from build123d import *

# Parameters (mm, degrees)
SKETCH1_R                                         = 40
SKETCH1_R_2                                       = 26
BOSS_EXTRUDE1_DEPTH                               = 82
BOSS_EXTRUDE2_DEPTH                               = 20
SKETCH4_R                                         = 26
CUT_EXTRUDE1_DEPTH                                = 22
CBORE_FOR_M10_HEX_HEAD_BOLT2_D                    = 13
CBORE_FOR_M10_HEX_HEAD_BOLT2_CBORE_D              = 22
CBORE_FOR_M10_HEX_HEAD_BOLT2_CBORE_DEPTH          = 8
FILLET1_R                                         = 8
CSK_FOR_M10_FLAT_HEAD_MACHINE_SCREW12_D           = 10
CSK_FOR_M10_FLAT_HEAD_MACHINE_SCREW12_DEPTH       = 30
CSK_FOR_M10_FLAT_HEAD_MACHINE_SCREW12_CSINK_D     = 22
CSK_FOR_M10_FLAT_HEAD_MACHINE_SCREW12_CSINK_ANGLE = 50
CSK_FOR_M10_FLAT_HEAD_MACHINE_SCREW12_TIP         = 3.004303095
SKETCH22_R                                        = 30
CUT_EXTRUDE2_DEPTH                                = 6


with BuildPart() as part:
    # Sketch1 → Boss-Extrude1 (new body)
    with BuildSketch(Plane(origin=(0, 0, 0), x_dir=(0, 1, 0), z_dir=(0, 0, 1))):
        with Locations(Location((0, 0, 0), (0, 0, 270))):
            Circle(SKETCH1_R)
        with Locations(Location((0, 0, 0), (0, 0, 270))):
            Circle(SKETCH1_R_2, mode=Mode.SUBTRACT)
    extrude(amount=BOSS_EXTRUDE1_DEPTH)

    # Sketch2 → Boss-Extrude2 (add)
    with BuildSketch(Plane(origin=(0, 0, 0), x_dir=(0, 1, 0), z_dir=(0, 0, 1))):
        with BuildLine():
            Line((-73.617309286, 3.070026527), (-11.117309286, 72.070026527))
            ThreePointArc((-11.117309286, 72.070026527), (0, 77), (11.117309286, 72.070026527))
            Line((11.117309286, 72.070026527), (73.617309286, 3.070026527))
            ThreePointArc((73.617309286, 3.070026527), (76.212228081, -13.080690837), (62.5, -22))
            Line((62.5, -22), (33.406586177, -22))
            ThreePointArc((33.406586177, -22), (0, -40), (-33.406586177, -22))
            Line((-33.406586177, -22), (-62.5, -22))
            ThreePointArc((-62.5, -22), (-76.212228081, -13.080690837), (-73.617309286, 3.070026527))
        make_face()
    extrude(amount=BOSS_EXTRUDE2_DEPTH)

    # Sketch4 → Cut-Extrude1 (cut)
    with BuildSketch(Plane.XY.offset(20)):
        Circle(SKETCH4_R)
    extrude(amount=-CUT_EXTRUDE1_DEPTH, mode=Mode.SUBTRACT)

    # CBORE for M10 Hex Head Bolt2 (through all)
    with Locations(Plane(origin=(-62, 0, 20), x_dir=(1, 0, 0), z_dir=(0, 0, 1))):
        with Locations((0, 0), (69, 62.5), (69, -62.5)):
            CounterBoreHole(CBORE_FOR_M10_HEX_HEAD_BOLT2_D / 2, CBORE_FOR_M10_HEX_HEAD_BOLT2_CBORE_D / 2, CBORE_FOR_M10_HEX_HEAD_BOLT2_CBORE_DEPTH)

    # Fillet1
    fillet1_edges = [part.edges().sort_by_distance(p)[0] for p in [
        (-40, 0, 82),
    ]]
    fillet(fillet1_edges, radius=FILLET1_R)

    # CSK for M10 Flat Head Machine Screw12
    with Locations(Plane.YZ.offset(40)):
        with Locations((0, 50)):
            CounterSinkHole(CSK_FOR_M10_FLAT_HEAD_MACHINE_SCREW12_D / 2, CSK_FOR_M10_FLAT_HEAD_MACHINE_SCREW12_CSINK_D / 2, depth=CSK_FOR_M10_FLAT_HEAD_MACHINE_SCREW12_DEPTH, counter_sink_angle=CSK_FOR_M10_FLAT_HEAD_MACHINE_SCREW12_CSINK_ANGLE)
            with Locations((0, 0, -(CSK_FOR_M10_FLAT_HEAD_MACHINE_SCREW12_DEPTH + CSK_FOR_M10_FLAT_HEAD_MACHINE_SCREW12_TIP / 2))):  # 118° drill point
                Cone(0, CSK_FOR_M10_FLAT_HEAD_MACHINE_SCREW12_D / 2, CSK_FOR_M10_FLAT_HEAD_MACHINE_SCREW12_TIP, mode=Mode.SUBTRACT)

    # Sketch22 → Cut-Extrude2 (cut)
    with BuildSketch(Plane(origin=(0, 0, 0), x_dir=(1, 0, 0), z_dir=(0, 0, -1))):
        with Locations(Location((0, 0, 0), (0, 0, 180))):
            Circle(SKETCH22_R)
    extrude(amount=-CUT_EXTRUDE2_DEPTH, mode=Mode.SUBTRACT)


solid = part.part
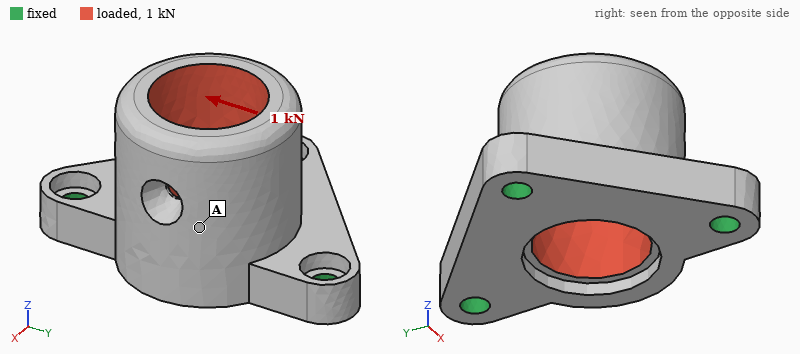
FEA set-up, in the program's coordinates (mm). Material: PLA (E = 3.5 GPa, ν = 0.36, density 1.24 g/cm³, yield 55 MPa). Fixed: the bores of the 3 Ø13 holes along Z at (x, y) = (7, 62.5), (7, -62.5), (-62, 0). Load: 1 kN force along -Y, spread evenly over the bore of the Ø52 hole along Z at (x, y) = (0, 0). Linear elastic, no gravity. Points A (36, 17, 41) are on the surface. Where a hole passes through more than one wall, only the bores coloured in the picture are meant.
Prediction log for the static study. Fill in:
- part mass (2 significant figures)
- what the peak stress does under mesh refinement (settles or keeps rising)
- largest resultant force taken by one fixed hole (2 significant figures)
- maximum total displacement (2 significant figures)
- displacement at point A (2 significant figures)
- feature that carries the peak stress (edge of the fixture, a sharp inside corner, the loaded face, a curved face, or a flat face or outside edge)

400 g
keeps rising
550 N
55 µm
28 µm
edge of the fixture
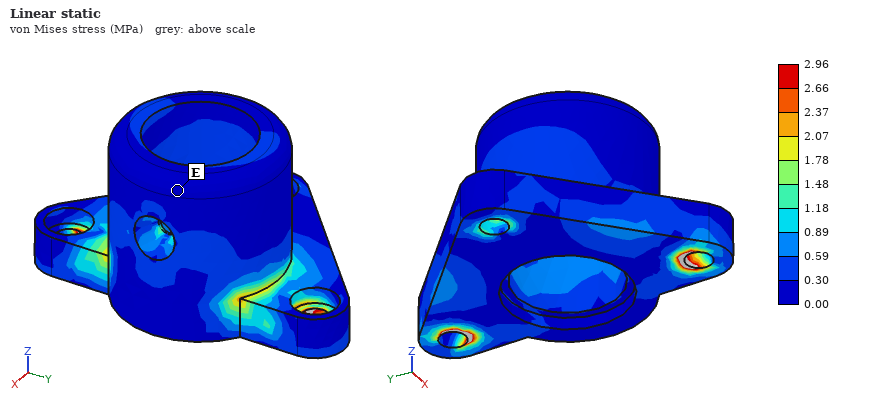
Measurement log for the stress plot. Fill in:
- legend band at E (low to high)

0.00 to 0.30 MPa
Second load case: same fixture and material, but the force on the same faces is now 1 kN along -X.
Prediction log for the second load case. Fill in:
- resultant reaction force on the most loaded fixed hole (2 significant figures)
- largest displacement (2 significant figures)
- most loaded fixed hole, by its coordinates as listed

800 N
0.15 mm
(-62, 0)
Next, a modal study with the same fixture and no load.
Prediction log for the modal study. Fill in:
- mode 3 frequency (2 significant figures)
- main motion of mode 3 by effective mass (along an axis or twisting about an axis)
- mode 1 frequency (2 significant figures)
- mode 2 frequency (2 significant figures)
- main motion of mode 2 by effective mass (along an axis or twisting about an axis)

1800 Hz
along Z
910 Hz
1500 Hz
along Y
